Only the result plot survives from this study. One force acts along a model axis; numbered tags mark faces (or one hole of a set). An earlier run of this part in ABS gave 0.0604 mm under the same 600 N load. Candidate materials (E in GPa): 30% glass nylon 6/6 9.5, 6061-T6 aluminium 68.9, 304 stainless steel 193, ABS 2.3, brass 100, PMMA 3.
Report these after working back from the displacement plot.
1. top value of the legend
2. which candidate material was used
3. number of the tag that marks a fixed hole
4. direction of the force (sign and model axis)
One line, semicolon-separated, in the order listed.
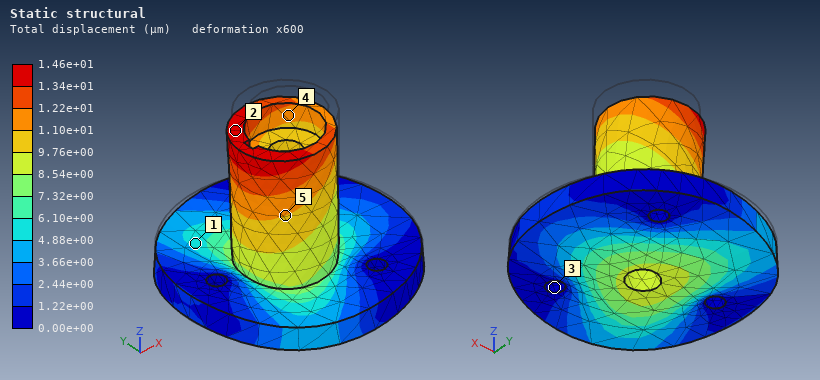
1.46e+01 µm; 30% glass nylon 6/6; 3; -Z
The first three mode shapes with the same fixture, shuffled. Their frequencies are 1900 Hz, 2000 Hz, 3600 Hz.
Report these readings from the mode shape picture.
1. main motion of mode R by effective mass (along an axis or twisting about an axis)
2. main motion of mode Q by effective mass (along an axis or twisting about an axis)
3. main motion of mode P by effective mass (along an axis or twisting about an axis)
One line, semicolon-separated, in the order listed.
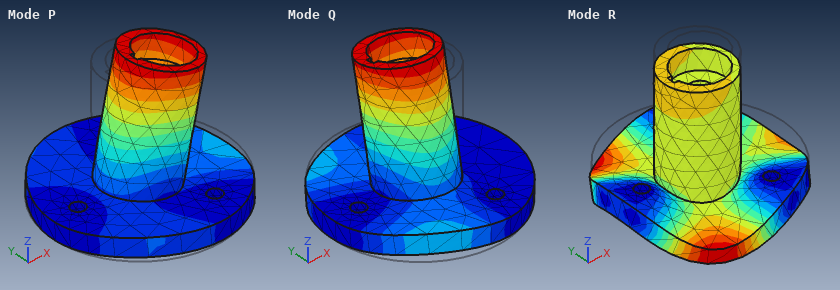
along Z; along Y; along X
